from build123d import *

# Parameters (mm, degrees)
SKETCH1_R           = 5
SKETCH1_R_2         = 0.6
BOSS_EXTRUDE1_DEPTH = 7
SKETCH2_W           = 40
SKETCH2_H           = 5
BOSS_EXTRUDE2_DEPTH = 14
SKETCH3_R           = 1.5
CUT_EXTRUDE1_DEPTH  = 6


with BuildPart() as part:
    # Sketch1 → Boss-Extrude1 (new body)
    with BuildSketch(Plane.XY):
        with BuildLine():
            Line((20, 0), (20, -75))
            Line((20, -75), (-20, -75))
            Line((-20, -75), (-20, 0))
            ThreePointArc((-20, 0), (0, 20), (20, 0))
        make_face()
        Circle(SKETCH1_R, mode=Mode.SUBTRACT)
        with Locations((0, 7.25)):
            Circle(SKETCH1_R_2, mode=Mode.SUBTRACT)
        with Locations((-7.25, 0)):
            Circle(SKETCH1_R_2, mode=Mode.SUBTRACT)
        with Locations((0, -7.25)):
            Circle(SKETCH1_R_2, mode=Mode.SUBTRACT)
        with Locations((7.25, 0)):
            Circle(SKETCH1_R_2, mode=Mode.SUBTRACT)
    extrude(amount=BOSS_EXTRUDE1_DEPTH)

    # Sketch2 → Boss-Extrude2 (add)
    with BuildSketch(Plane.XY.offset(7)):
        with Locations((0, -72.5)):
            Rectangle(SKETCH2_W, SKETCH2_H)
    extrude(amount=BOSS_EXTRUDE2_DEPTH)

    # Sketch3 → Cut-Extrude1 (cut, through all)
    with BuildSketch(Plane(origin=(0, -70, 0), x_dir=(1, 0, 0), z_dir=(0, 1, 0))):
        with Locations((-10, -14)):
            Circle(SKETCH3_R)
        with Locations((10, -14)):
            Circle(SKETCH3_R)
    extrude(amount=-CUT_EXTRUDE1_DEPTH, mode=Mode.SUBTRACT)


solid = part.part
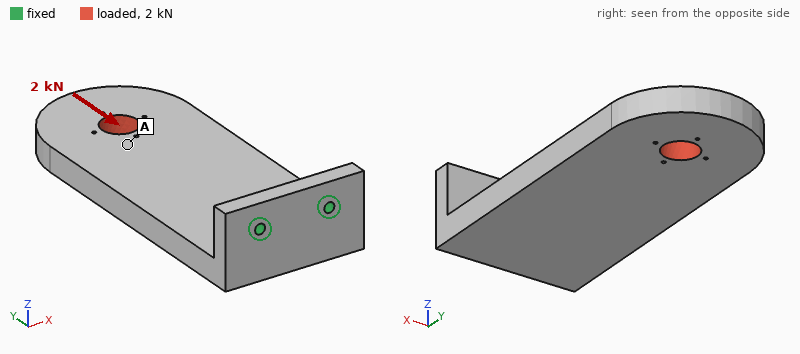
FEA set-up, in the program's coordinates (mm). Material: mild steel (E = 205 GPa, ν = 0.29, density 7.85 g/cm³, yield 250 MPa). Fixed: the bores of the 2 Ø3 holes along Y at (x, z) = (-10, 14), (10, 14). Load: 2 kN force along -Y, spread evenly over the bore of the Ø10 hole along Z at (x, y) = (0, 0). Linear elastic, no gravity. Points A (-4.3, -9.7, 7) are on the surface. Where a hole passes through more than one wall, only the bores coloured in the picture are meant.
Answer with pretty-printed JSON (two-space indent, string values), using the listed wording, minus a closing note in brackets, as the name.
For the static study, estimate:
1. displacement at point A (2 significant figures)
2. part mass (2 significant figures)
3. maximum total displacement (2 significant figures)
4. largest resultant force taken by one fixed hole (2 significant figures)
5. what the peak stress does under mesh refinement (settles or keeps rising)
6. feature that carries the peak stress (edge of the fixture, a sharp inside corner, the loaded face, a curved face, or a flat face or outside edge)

{
  "displacement at point A": "0.10 mm",
  "part mass": "220 g",
  "maximum total displacement": "0.15 mm",
  "largest resultant force taken by one fixed hole": "1.0 kN",
  "what the peak stress does under mesh refinement": "keeps rising",
  "feature that carries the peak stress": "edge of the fixture"
}
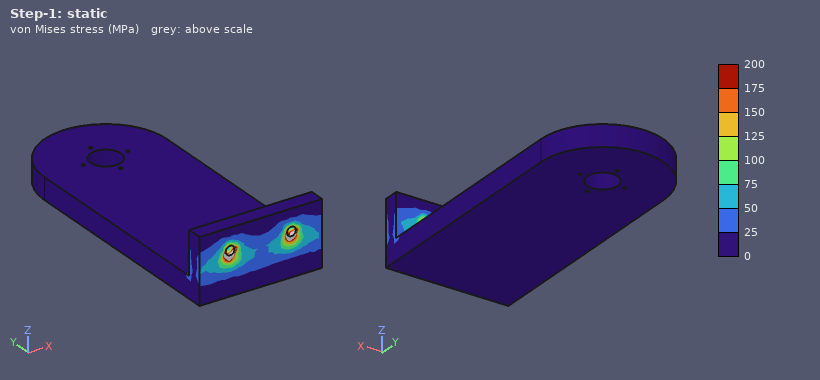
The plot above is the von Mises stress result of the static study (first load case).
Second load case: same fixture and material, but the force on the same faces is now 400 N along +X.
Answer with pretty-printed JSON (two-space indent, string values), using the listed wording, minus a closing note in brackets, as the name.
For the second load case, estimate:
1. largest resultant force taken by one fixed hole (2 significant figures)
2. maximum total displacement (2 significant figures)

{
  "largest resultant force taken by one fixed hole": "1.2 kN",
  "maximum total displacement": "67 µm"
}
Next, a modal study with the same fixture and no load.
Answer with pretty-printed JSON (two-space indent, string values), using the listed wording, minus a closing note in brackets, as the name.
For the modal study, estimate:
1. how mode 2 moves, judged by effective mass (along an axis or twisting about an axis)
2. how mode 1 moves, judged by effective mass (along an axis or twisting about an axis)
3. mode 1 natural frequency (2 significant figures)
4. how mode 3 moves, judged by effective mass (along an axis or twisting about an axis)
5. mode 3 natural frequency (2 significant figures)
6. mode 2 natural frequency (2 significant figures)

{
  "how mode 2 moves, judged by effective mass": "along X",
  "how mode 1 moves, judged by effective mass": "along Z",
  "mode 1 natural frequency": "500 Hz",
  "how mode 3 moves, judged by effective mass": "twisting about Y",
  "mode 3 natural frequency": "3300 Hz",
  "mode 2 natural frequency": "1400 Hz"
}
